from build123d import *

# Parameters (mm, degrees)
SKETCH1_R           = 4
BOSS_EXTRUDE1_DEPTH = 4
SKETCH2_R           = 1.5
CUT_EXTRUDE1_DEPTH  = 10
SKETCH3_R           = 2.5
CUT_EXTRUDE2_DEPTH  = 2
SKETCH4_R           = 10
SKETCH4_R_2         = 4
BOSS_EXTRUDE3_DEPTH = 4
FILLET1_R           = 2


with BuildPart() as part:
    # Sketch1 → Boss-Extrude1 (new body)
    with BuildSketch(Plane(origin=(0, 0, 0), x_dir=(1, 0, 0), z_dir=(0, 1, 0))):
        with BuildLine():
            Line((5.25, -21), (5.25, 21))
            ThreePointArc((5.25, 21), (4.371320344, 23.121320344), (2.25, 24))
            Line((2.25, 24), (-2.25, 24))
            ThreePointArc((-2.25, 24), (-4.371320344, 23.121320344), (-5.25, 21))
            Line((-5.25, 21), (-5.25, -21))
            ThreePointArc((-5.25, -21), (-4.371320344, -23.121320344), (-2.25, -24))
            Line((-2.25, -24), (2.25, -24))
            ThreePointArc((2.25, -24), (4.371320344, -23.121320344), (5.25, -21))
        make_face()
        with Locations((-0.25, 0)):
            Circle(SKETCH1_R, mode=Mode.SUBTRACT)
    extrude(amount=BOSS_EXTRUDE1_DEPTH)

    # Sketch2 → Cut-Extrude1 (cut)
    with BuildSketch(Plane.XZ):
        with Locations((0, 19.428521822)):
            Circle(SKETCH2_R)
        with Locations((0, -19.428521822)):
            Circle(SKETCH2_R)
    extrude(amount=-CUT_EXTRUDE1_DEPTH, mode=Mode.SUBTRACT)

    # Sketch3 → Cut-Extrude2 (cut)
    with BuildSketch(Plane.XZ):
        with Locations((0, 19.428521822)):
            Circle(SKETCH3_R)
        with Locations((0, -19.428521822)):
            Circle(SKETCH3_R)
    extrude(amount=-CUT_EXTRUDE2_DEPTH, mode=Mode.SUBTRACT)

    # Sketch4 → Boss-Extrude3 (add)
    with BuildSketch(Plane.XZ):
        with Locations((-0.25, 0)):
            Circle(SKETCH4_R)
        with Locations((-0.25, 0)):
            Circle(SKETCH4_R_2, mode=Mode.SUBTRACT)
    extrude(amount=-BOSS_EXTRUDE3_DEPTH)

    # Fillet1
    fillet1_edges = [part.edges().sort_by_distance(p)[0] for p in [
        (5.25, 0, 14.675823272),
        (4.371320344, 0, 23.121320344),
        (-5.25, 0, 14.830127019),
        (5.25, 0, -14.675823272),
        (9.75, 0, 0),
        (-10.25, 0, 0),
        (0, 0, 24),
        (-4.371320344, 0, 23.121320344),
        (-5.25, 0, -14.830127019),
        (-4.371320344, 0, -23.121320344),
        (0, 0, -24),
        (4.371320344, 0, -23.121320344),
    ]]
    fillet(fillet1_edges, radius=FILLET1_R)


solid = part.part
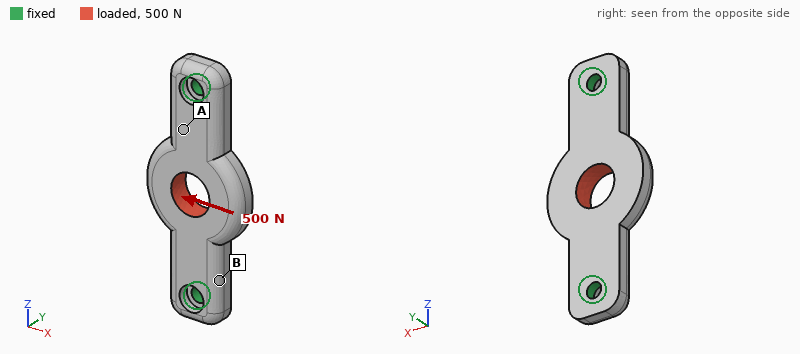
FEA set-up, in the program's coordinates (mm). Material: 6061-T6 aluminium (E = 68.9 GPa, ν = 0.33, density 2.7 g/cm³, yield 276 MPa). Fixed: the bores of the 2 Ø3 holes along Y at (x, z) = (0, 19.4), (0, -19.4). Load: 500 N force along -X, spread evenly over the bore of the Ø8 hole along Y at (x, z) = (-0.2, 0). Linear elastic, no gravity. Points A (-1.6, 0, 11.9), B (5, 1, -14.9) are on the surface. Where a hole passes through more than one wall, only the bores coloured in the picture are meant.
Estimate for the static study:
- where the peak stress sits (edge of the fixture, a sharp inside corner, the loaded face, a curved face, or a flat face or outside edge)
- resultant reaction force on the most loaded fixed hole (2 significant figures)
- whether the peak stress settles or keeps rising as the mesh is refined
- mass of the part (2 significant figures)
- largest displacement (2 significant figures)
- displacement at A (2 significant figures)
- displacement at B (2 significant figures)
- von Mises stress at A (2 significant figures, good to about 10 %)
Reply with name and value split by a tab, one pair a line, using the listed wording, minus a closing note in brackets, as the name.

where the peak stress sits	edge of the fixture
resultant reaction force on the most loaded fixed hole	250 N
whether the peak stress settles or keeps rising as the mesh is refined	keeps rising
mass of the part	5.5 g
largest displacement	12 µm
displacement at A	7.7 µm
displacement at B	5.9 µm
von Mises stress at A	15 MPa
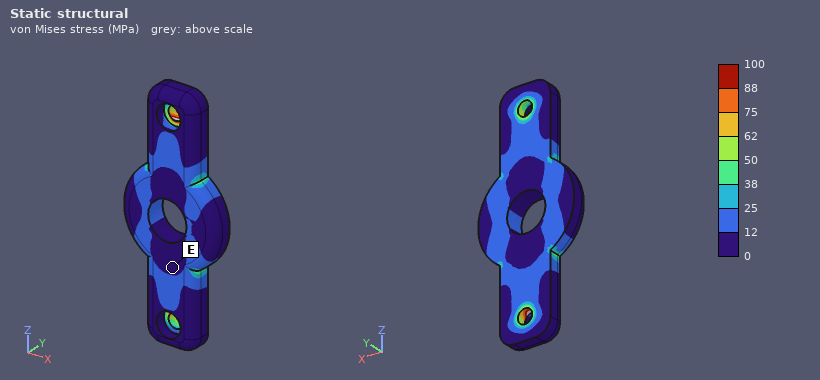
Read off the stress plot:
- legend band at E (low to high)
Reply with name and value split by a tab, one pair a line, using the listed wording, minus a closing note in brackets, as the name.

legend band at E	0 to 12 MPa
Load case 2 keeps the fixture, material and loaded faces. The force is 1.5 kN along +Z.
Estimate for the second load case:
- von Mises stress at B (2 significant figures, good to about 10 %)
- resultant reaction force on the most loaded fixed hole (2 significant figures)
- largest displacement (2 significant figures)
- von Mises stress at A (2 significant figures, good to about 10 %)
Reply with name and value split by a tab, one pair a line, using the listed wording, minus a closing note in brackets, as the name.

von Mises stress at B	10 MPa
resultant reaction force on the most loaded fixed hole	750 N
largest displacement	7.2 µm
von Mises stress at A	9.1 MPa
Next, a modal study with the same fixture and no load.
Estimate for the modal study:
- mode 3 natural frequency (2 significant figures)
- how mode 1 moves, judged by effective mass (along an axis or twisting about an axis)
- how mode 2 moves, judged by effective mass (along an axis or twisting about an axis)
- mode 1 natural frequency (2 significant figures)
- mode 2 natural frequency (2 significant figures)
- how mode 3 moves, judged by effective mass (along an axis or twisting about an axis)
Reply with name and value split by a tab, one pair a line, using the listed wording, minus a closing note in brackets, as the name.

mode 3 natural frequency	20 kHz
how mode 1 moves, judged by effective mass	along Y
how mode 2 moves, judged by effective mass	twisting about Z
mode 1 natural frequency	9000 Hz
mode 2 natural frequency	12 kHz
how mode 3 moves, judged by effective mass	along X
